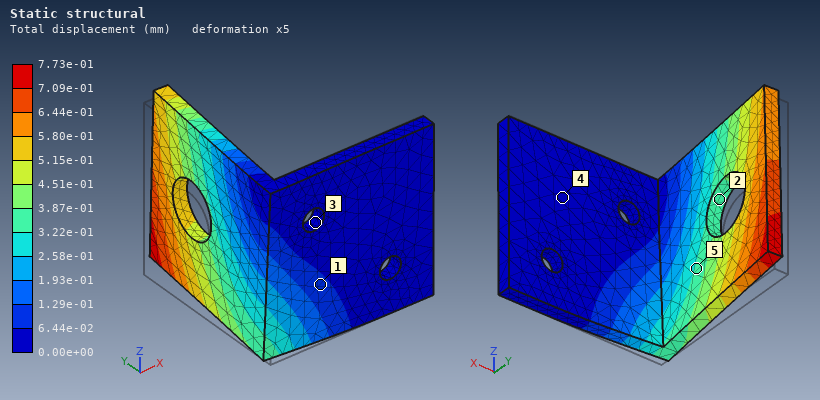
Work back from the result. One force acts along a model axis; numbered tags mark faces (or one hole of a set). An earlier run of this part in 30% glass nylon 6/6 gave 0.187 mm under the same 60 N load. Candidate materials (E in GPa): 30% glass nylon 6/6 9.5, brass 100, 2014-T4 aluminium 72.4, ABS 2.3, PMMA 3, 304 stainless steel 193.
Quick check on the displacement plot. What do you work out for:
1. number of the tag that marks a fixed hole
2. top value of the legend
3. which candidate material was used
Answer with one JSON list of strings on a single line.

["3", "7.73e-01 mm", "ABS"]
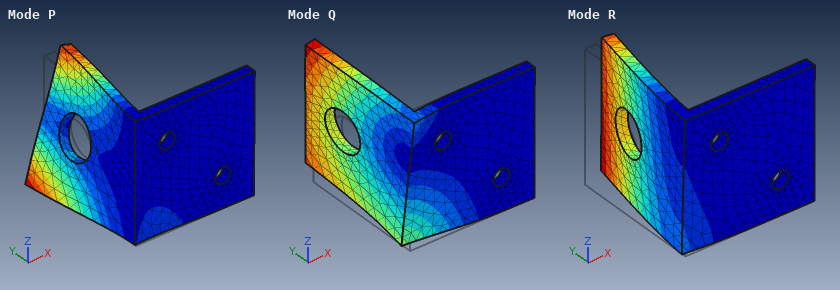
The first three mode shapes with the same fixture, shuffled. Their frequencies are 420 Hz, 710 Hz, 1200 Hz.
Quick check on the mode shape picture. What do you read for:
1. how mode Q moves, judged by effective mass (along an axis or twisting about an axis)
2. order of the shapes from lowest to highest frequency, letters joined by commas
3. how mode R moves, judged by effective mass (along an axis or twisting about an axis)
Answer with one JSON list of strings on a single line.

["along Z", "R, Q, P", "along X"]
